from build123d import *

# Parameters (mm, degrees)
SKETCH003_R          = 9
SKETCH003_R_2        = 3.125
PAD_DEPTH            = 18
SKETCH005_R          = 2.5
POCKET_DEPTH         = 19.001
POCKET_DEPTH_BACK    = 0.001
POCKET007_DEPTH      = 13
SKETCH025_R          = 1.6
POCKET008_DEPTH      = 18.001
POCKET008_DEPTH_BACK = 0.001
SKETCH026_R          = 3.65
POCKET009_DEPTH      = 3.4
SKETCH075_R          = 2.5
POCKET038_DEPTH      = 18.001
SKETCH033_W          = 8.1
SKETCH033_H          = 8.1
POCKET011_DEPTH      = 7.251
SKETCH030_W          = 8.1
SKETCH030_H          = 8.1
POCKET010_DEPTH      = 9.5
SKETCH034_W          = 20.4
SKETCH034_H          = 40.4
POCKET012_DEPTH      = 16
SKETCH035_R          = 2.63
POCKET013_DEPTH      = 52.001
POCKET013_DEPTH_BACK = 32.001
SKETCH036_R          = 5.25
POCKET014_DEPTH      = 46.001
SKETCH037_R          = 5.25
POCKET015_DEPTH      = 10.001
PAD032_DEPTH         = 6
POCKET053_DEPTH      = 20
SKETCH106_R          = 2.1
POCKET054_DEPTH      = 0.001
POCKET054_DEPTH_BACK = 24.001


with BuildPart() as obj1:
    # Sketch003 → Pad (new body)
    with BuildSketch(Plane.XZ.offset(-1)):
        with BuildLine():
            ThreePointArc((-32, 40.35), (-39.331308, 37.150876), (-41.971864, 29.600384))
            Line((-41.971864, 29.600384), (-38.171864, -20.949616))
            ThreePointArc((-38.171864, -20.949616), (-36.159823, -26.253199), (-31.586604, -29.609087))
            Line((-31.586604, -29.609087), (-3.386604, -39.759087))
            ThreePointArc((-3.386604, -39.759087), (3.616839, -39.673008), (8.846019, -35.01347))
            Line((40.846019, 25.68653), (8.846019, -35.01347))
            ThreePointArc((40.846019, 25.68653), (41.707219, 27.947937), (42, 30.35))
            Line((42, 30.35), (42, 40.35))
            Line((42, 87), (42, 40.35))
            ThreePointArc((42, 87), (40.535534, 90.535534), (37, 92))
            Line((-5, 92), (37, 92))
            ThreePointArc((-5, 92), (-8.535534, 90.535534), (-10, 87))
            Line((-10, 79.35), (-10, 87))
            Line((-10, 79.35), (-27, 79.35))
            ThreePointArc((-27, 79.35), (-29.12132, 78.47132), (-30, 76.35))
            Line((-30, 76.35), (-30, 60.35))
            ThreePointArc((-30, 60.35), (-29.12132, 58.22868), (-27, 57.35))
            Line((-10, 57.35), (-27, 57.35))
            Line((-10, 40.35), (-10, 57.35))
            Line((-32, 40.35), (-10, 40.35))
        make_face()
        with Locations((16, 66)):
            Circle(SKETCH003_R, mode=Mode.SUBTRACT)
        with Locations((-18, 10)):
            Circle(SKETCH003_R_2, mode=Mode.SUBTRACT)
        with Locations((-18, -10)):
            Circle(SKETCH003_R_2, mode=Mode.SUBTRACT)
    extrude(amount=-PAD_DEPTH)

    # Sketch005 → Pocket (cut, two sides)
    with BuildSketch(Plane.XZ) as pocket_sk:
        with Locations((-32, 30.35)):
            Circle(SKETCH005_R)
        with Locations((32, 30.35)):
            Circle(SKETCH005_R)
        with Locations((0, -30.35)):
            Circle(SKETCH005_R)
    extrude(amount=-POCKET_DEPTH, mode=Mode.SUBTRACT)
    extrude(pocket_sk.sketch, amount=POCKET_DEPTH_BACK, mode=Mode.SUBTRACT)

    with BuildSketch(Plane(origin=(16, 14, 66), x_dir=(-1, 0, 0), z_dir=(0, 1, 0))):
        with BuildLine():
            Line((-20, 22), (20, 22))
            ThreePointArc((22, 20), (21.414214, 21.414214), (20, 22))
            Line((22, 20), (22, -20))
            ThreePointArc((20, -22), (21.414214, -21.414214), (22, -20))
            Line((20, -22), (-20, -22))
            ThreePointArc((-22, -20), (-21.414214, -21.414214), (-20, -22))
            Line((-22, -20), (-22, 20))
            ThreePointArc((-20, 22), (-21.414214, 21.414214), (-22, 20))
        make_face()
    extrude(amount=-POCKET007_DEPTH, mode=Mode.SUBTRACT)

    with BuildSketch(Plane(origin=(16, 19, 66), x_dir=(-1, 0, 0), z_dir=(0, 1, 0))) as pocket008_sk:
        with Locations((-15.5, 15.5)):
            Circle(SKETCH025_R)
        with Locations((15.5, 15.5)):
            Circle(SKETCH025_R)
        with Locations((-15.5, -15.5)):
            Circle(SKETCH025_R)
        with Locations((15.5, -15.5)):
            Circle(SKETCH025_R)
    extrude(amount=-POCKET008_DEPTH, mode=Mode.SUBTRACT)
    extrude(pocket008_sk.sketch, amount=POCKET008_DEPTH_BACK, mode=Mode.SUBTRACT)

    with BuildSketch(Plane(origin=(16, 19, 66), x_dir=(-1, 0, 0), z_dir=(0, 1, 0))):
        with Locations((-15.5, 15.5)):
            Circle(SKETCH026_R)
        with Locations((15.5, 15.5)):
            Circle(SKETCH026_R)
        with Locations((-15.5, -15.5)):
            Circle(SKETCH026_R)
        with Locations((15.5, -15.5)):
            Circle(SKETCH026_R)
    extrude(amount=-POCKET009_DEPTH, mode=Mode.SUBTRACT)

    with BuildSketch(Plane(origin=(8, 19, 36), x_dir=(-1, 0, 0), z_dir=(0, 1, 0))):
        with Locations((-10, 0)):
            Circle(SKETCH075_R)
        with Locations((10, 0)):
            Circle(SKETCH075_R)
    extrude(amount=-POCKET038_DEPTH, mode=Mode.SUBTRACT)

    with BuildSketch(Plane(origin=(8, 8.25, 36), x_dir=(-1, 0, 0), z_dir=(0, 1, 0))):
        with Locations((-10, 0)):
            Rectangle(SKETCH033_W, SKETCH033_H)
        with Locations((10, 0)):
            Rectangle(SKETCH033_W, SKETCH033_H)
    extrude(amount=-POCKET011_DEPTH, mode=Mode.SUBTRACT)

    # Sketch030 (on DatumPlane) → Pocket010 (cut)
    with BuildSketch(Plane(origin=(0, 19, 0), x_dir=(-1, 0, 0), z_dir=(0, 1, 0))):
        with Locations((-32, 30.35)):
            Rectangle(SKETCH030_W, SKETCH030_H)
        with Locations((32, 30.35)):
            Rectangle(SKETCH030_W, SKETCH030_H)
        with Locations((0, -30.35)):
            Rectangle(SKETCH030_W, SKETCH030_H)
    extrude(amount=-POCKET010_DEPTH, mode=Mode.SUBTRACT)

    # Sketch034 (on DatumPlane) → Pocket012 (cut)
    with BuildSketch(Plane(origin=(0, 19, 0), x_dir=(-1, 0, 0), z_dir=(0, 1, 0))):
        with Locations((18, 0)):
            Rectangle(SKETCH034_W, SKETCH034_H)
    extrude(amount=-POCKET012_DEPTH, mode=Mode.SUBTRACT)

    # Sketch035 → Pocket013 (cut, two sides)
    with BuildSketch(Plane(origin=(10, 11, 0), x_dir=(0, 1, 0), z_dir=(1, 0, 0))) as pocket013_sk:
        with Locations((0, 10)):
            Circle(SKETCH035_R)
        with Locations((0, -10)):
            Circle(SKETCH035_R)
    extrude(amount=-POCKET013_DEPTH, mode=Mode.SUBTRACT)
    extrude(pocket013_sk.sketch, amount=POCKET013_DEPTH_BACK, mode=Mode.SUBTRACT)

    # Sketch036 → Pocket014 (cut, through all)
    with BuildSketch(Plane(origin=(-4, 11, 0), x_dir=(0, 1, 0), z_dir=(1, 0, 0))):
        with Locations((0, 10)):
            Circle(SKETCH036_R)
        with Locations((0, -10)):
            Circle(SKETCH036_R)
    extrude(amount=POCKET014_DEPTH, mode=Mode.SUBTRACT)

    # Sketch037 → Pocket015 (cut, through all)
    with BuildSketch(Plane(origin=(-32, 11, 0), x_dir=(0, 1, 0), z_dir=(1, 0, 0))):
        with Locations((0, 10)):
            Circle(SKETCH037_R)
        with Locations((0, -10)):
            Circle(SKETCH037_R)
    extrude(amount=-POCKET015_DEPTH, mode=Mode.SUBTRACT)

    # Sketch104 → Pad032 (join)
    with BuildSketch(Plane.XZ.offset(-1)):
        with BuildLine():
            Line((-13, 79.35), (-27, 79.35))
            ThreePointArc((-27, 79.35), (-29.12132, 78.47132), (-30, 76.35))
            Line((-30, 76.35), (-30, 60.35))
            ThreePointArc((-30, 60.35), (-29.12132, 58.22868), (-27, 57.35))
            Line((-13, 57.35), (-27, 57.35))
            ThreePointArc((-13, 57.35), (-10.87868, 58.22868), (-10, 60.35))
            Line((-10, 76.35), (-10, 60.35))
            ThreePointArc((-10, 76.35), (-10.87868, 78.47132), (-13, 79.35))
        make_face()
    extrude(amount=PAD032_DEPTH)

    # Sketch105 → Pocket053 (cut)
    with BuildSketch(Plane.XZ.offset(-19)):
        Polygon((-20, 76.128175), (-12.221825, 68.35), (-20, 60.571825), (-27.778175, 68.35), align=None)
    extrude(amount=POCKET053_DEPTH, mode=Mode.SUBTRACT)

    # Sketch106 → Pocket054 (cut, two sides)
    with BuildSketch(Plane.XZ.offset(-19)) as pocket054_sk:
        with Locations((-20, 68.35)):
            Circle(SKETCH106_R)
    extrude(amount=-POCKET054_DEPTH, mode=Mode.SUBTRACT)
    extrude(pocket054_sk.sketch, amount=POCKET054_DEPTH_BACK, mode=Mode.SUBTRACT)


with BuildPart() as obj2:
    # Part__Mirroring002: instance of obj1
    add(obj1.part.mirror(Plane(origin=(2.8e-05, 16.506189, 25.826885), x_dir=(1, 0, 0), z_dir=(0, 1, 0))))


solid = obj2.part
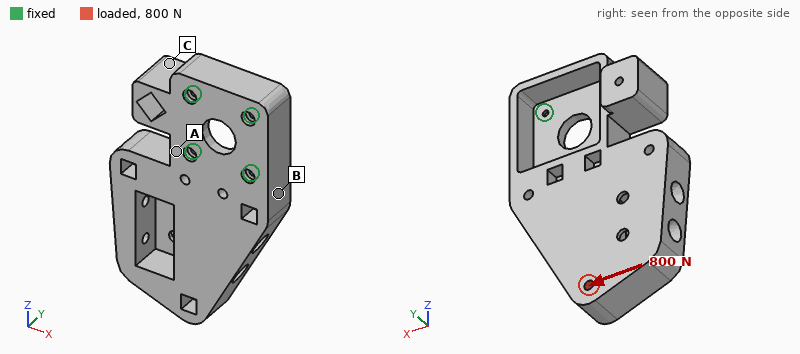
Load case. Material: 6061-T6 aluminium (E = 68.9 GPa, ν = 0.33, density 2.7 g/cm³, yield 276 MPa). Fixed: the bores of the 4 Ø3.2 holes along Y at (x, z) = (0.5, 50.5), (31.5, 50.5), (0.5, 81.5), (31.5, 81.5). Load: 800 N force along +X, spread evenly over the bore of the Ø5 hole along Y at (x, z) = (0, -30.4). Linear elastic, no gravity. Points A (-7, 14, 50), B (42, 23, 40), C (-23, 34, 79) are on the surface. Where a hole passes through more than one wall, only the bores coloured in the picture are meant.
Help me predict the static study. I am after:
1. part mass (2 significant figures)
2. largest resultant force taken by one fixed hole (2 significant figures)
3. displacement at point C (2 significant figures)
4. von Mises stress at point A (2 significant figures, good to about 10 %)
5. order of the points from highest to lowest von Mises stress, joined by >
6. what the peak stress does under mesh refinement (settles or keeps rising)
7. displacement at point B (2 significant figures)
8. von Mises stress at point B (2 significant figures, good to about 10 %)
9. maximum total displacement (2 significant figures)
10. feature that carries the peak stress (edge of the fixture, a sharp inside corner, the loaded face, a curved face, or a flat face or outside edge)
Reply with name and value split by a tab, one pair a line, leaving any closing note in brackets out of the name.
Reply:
part mass	260 g
largest resultant force taken by one fixed hole	1.3 kN
displacement at point C	9.7 µm
von Mises stress at point A	14 MPa
order of the points from highest to lowest von Mises stress, joined by >	A > B > C
what the peak stress does under mesh refinement	keeps rising
displacement at point B	11 µm
von Mises stress at point B	9.4 MPa
maximum total displacement	51 µm
feature that carries the peak stress	edge of the fixture
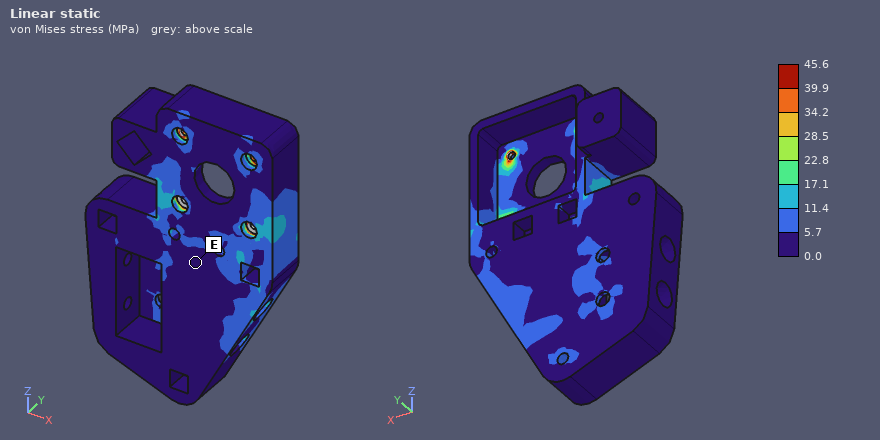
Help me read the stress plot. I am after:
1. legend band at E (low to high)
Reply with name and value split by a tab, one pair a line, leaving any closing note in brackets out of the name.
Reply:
legend band at E	0.0 to 5.7 MPa
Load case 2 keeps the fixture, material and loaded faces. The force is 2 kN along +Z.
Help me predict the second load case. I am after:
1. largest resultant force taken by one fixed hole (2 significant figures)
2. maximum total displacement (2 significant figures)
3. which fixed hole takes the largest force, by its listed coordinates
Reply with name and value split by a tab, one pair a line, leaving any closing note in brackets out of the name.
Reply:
largest resultant force taken by one fixed hole	1.2 kN
maximum total displacement	0.15 mm
which fixed hole takes the largest force, by its listed coordinates	(0.5, 50.5)
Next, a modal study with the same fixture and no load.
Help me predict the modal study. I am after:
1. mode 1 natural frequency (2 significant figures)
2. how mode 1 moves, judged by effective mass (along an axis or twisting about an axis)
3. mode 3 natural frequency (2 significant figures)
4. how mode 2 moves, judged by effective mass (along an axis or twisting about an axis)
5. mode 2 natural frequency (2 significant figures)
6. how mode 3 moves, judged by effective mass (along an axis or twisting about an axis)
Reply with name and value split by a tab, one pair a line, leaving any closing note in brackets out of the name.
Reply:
mode 1 natural frequency	790 Hz
how mode 1 moves, judged by effective mass	along Y
mode 3 natural frequency	2400 Hz
how mode 2 moves, judged by effective mass	twisting about Z
mode 2 natural frequency	2300 Hz
how mode 3 moves, judged by effective mass	along X
